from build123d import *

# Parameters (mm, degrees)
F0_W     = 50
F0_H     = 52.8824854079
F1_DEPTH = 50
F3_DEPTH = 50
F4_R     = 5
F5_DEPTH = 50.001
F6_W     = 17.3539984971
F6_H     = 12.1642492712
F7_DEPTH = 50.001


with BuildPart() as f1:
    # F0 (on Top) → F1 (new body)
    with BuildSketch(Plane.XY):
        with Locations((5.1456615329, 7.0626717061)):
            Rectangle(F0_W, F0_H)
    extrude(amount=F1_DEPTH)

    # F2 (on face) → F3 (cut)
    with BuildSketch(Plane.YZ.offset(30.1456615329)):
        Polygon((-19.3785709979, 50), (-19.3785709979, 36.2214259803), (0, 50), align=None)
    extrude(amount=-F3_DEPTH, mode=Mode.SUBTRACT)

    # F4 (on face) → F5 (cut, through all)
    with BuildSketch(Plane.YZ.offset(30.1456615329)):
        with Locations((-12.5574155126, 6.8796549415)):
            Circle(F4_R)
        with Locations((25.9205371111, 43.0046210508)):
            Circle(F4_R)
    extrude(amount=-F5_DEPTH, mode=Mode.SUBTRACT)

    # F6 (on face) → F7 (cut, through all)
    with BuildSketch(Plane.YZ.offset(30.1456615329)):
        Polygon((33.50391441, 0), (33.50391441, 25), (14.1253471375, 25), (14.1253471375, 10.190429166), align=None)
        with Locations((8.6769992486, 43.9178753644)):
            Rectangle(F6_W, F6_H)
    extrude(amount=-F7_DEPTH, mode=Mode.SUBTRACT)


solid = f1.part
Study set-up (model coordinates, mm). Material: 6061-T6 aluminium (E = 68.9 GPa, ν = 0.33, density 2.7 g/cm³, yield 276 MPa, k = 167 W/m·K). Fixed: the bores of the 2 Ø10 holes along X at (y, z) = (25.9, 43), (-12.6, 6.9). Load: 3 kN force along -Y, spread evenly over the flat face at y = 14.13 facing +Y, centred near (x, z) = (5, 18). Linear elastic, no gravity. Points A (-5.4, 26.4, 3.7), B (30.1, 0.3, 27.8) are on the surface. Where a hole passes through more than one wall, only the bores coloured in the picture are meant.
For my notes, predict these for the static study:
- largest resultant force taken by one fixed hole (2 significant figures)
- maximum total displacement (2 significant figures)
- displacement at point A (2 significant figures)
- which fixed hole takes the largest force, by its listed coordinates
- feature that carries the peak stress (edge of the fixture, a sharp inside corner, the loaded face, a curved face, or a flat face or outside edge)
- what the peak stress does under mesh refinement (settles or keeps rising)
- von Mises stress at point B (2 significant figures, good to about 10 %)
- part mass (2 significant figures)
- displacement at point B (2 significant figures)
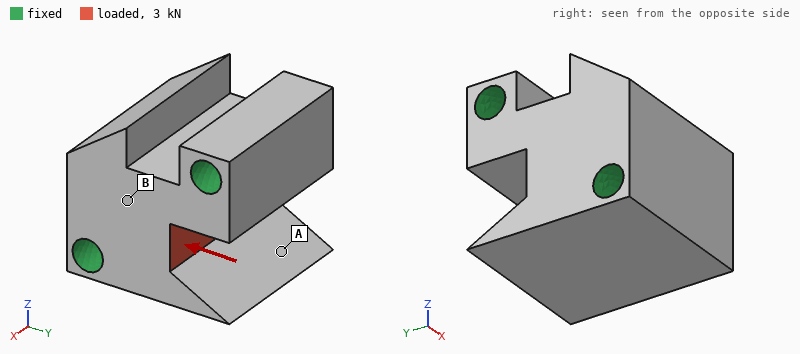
2.0 kN
2.4 µm
1.9 µm
(-12.6, 6.9)
edge of the fixture
keeps rising
1.7 MPa
240 g
1.1 µm
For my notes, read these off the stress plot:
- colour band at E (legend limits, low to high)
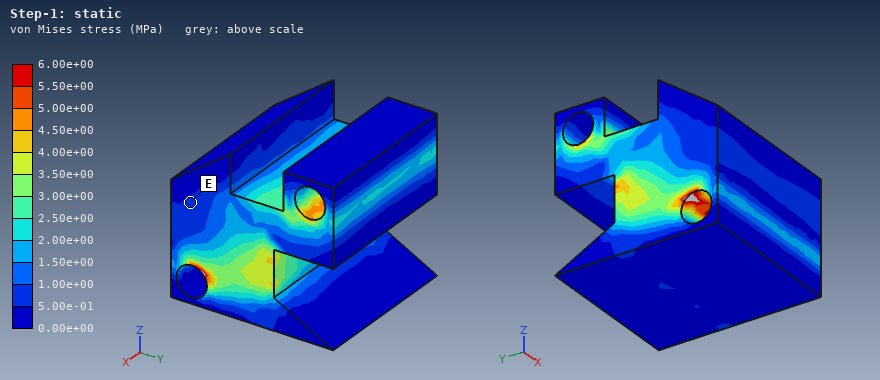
5.00e-01 to 1.00e+00 MPa
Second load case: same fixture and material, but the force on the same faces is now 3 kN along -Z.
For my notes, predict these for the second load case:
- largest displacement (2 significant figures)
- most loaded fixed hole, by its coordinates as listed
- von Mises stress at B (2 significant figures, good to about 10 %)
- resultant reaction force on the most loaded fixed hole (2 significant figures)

5.0 µm
(-12.6, 6.9)
2.9 MPa
1.9 kN
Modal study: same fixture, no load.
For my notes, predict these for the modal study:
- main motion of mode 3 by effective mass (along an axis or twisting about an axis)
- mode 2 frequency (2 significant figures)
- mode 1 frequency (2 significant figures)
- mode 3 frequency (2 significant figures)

along X
17 kHz
14 kHz
21 kHz
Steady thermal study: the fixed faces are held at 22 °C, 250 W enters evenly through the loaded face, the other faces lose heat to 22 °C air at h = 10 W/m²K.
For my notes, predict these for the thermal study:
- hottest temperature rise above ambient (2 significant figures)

25 K
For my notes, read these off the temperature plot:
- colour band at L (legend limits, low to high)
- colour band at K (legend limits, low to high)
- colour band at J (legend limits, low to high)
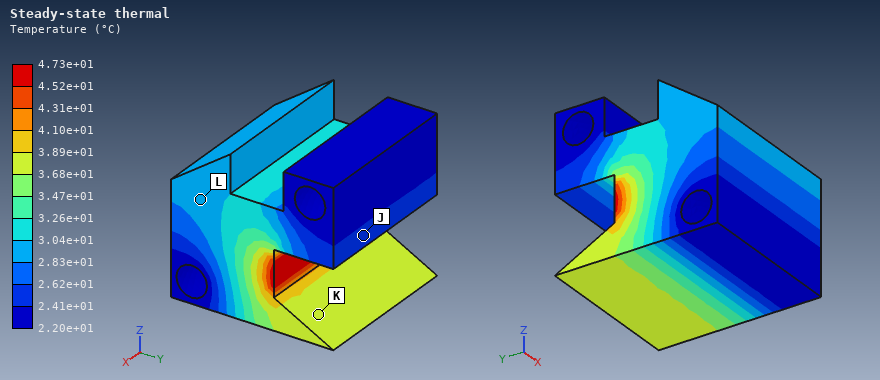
2.83e+01 to 3.04e+01 °C
3.68e+01 to 3.89e+01 °C
2.41e+01 to 2.62e+01 °C
